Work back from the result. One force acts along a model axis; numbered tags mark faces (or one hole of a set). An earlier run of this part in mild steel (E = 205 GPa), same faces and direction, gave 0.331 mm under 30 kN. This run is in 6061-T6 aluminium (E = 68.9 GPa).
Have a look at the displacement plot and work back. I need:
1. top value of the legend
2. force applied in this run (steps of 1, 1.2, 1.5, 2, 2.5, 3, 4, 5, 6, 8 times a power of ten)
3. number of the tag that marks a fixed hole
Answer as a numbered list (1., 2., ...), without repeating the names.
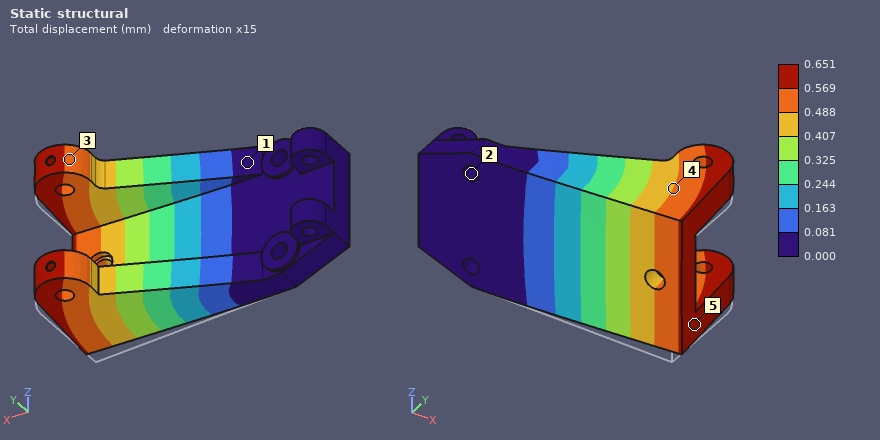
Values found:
1. 0.651 mm
2. 20 kN
3. 2
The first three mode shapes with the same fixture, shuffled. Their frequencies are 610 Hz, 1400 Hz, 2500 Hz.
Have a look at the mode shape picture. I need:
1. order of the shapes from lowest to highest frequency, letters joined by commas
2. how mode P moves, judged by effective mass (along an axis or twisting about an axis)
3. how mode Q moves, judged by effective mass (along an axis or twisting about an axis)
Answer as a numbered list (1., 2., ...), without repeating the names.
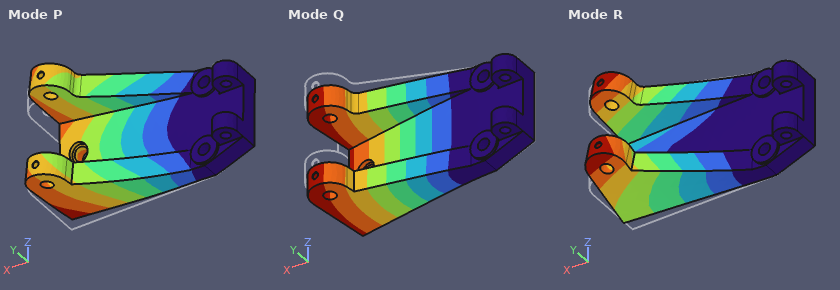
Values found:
1. Q, R, P
2. along Z
3. along Y
